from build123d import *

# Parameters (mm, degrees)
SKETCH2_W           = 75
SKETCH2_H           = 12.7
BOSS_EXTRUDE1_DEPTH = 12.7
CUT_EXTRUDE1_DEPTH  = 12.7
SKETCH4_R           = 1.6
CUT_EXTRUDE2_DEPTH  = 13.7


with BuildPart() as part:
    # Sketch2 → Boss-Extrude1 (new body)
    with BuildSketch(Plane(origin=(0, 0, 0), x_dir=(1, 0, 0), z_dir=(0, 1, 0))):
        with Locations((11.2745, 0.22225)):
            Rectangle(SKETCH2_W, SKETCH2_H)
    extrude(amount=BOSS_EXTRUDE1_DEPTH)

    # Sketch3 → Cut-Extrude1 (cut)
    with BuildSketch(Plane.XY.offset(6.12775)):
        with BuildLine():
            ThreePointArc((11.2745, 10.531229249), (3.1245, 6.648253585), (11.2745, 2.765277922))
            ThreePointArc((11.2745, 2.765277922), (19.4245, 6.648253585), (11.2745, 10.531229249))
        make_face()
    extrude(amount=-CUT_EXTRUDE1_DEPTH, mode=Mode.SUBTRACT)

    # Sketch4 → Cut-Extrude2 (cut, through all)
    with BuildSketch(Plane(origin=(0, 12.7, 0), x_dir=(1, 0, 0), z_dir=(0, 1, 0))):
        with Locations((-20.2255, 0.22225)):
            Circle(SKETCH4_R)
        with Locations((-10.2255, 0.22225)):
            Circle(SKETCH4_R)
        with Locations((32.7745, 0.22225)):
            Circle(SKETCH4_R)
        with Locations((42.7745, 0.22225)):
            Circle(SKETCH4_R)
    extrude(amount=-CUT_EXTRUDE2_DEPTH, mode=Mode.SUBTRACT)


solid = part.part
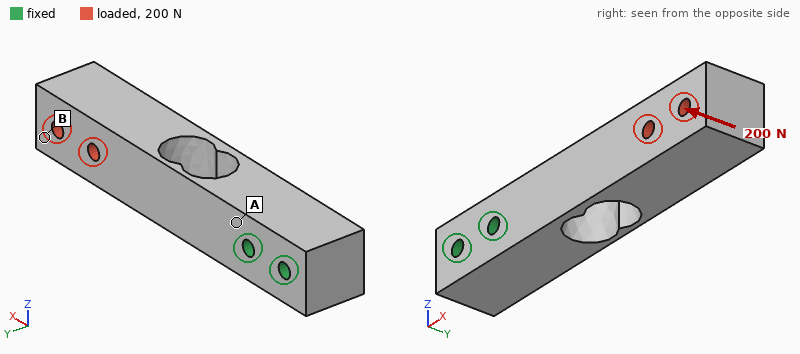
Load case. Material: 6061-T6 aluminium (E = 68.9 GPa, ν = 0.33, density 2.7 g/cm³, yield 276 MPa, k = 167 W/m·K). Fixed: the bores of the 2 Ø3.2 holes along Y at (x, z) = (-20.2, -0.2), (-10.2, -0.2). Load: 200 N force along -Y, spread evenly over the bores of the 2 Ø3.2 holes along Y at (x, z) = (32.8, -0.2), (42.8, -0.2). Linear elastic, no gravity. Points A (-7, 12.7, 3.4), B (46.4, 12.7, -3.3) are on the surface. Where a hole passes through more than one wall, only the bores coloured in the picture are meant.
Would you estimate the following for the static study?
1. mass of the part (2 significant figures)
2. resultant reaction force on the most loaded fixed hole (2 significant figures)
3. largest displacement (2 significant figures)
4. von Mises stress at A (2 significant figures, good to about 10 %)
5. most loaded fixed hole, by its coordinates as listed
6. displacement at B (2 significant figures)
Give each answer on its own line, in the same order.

27 g
340 N
0.16 mm
22 MPa
(-10.2, -0.2)
0.15 mm
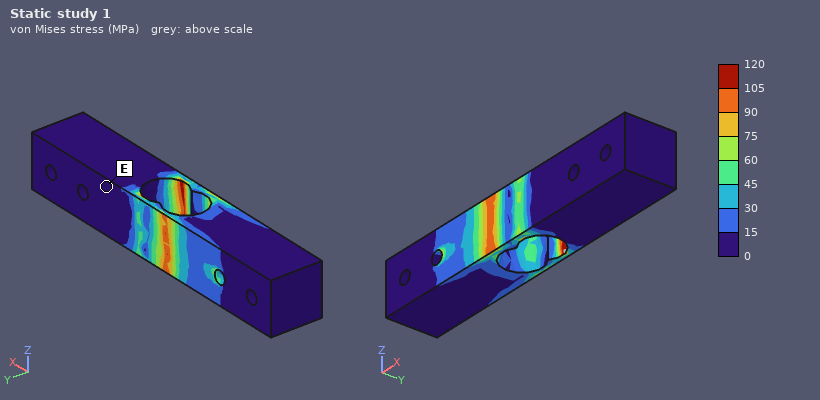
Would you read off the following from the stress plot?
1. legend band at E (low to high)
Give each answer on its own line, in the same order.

0 to 15 MPa
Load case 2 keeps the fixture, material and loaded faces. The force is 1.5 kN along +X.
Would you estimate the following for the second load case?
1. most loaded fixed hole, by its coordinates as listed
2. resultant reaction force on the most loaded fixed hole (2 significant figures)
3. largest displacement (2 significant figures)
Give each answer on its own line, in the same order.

(-10.2, -0.2)
1.3 kN
22 µm
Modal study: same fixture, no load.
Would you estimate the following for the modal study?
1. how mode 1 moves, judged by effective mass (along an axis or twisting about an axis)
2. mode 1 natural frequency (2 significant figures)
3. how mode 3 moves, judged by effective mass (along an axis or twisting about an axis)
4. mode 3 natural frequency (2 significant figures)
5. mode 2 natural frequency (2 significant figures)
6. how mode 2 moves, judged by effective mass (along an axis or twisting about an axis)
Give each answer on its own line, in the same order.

along Y
1800 Hz
twisting about X
7400 Hz
1900 Hz
along Z
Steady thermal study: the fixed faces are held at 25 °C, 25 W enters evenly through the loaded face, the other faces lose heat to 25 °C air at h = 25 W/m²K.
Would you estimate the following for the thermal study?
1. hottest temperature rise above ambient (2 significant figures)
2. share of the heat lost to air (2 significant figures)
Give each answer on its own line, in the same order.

76 K
16 %
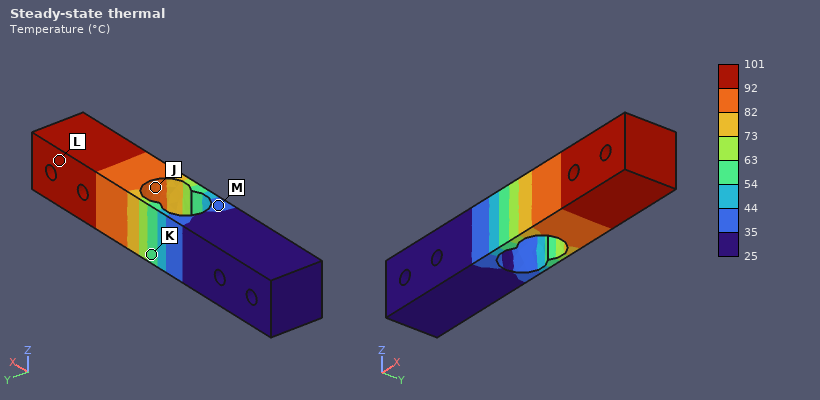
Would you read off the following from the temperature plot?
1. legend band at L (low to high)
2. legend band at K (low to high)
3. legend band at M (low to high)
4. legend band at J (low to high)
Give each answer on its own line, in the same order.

92 to 101 °C
54 to 63 °C
35 to 44 °C
82 to 92 °C
